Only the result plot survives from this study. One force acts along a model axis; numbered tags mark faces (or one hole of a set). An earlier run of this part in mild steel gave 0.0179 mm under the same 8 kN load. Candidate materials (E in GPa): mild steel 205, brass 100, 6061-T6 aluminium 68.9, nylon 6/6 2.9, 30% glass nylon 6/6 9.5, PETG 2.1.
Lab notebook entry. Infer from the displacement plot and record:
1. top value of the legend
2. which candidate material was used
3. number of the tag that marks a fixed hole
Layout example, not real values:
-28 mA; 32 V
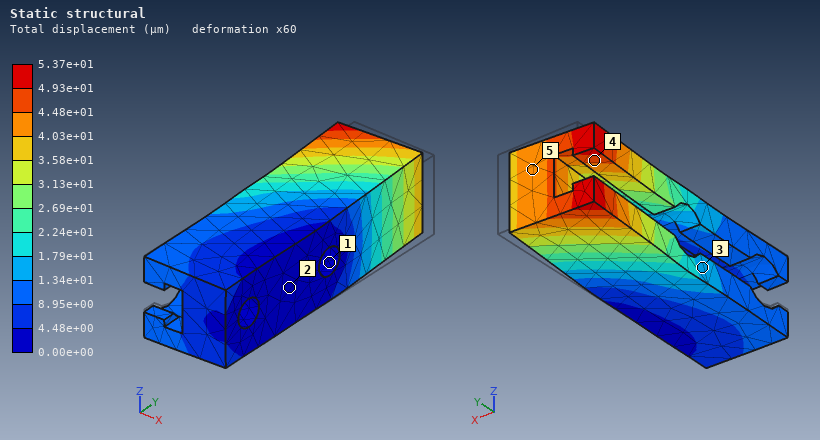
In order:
5.37e+01 µm; 6061-T6 aluminium; 1
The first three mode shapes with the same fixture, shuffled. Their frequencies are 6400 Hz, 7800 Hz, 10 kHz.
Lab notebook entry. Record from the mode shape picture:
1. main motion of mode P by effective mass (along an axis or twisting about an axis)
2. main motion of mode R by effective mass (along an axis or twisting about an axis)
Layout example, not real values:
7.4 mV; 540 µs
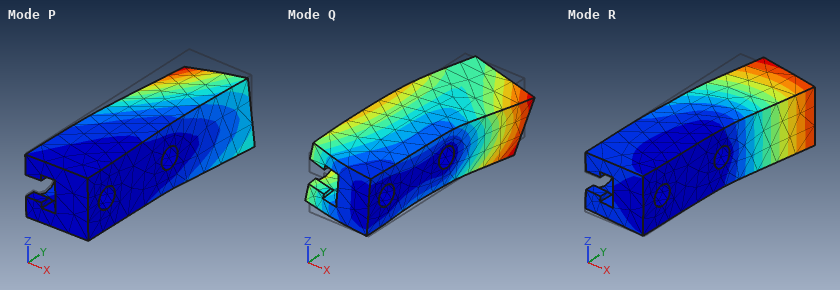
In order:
along Z; along X
